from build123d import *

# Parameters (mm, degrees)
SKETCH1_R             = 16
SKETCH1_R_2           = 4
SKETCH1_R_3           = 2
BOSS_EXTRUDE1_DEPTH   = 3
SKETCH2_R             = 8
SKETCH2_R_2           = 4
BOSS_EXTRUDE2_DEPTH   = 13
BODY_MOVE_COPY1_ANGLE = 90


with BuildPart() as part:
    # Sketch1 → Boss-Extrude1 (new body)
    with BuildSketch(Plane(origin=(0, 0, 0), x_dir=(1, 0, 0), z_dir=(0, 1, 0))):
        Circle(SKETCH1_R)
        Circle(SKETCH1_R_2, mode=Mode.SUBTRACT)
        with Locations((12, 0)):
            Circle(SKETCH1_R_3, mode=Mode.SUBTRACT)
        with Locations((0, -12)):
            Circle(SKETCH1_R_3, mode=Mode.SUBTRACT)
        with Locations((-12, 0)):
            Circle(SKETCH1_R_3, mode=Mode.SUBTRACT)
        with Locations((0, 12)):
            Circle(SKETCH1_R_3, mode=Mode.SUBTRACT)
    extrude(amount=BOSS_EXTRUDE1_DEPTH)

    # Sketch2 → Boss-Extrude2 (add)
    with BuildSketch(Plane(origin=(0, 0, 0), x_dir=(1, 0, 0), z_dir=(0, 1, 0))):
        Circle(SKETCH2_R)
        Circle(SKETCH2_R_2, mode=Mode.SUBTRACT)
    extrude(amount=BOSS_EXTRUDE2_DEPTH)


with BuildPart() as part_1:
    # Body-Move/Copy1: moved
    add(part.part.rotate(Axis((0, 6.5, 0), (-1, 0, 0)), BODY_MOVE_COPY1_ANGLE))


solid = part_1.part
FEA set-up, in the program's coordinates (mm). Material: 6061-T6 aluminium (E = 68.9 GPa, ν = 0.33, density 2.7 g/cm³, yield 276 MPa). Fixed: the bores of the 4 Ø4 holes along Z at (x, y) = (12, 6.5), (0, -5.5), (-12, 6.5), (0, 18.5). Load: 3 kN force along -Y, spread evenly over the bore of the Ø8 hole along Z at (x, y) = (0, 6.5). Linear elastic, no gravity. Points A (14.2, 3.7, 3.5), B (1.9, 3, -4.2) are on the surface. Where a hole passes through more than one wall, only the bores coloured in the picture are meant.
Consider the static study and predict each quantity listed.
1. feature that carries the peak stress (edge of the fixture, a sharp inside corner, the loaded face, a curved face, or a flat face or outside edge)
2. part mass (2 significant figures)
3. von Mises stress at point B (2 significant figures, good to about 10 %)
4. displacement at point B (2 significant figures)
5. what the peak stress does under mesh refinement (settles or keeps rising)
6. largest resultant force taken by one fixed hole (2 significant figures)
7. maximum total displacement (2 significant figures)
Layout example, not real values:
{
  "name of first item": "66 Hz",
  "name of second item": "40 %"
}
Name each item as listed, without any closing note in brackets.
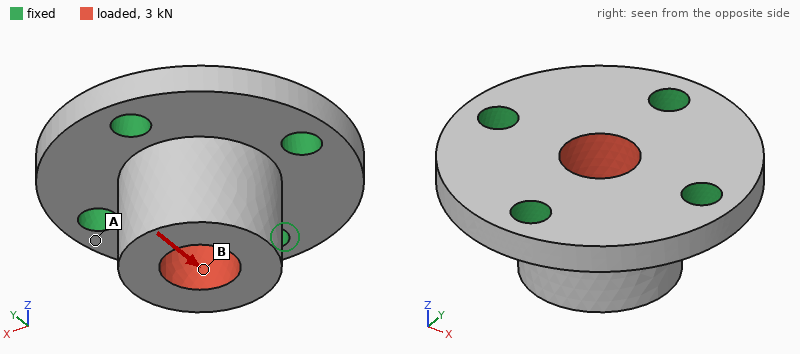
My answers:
{
  "feature that carries the peak stress": "edge of the fixture",
  "part mass": "9.8 g",
  "von Mises stress at point B": "18 MPa",
  "displacement at point B": "15 µm",
  "what the peak stress does under mesh refinement": "keeps rising",
  "largest resultant force taken by one fixed hole": "1.2 kN",
  "maximum total displacement": "18 µm"
}
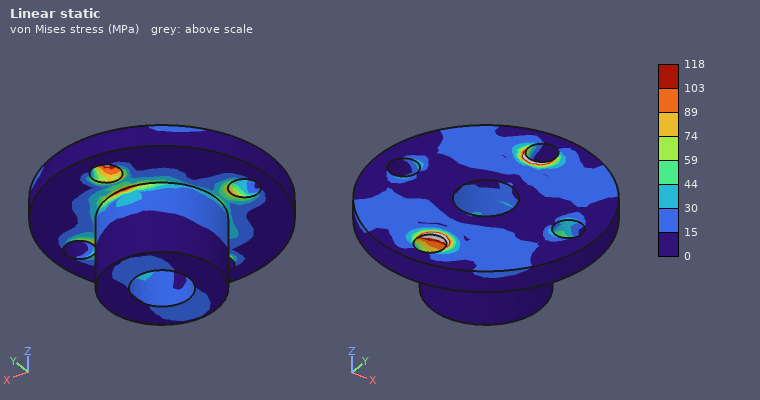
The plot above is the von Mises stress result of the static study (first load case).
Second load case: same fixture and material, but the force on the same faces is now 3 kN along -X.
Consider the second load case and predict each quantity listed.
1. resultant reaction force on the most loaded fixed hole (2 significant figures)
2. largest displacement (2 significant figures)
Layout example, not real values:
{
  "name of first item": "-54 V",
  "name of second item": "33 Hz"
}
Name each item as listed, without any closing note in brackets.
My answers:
{
  "resultant reaction force on the most loaded fixed hole": "1.2 kN",
  "largest displacement": "19 µm"
}
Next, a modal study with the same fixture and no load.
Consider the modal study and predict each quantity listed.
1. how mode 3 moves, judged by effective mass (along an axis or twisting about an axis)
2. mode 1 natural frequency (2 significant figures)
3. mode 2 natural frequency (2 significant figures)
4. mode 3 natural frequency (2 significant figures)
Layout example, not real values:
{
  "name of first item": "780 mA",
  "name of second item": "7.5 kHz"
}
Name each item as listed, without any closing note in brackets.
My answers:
{
  "how mode 3 moves, judged by effective mass": "along Z",
  "mode 1 natural frequency": "31 kHz",
  "mode 2 natural frequency": "31 kHz",
  "mode 3 natural frequency": "38 kHz"
}
